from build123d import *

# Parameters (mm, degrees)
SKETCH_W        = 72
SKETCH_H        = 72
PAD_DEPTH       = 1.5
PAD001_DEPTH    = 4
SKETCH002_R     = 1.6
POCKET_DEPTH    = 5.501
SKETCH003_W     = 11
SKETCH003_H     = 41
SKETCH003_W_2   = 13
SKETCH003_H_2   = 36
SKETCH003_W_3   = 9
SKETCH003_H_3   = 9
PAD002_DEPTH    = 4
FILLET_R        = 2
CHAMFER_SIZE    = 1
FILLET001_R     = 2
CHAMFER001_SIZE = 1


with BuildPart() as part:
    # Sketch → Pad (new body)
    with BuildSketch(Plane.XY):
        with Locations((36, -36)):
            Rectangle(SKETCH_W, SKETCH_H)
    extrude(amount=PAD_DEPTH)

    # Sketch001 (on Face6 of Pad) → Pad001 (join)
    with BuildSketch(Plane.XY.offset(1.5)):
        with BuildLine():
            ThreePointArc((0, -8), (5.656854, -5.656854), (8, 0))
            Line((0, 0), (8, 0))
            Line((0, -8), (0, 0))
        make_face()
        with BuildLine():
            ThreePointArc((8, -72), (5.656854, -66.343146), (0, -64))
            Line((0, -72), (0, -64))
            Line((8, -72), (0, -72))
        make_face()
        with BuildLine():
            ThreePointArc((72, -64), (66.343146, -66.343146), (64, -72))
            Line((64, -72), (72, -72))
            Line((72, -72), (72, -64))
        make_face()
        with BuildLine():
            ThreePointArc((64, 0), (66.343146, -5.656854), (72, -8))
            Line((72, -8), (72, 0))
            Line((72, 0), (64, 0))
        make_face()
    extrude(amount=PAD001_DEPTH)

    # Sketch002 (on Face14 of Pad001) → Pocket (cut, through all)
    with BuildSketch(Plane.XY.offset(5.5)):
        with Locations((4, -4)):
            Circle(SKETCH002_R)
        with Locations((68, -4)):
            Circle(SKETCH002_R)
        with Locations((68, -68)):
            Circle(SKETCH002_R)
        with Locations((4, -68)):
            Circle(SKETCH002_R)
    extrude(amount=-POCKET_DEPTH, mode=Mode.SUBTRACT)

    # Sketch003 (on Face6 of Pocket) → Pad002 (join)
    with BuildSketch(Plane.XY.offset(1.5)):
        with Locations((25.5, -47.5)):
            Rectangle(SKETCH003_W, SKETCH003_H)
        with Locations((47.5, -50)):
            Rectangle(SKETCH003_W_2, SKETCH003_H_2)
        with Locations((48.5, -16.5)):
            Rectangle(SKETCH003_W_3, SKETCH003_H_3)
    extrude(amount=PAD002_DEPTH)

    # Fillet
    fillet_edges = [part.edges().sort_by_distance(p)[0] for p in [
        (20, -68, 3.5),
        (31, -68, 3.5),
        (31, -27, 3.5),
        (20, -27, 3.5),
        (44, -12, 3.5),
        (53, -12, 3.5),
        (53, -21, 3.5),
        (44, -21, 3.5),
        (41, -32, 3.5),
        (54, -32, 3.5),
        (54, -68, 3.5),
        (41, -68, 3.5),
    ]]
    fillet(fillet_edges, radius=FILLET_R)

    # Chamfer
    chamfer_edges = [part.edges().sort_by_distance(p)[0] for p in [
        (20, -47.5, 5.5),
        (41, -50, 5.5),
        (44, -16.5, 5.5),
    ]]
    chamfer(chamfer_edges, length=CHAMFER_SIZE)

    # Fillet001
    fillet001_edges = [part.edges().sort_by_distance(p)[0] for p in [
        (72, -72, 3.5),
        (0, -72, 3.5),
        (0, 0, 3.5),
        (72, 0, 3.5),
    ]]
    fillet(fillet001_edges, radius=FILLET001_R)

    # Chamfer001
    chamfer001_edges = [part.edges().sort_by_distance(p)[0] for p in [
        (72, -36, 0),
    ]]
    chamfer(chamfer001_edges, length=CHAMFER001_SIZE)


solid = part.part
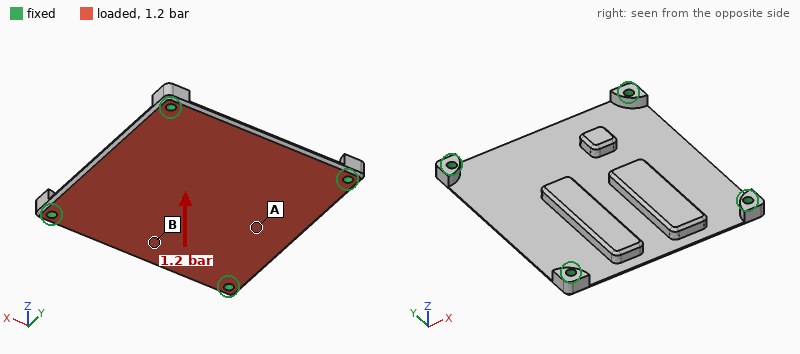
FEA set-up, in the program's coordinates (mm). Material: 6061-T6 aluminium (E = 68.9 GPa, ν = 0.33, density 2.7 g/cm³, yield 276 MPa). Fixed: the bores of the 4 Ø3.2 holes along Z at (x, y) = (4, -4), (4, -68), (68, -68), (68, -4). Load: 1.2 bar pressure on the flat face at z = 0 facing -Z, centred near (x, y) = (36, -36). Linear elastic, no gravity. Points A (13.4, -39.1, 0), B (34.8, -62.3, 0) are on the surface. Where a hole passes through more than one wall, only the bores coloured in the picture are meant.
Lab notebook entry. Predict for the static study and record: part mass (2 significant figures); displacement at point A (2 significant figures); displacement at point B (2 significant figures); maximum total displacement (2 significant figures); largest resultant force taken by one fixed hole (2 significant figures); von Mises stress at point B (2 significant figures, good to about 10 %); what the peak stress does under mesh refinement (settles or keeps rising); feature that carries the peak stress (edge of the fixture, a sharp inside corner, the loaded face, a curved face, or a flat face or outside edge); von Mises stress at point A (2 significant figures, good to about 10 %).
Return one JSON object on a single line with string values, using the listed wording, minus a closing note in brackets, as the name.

{"part mass": "33 g", "displacement at point A": "0.31 mm", "displacement at point B": "0.29 mm", "maximum total displacement": "0.50 mm", "largest resultant force taken by one fixed hole": "150 N", "von Mises stress at point B": "69 MPa", "what the peak stress does under mesh refinement": "keeps rising", "feature that carries the peak stress": "edge of the fixture", "von Mises stress at point A": "26 MPa"}
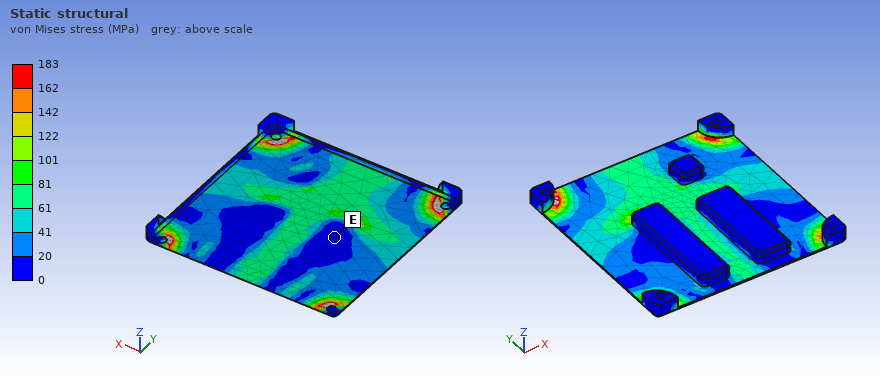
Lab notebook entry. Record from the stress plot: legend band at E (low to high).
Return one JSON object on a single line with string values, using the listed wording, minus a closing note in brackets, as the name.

{"legend band at E": "0 to 20 MPa"}
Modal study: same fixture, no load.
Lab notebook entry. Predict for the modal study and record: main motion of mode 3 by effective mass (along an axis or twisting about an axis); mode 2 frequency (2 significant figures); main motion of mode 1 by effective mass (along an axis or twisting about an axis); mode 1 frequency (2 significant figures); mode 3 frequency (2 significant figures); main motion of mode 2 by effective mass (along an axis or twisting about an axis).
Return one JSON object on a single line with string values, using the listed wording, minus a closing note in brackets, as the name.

{"main motion of mode 3 by effective mass": "twisting about Y", "mode 2 frequency": "2300 Hz", "main motion of mode 1 by effective mass": "along Z", "mode 1 frequency": "1200 Hz", "mode 3 frequency": "2600 Hz", "main motion of mode 2 by effective mass": "twisting about X"}
